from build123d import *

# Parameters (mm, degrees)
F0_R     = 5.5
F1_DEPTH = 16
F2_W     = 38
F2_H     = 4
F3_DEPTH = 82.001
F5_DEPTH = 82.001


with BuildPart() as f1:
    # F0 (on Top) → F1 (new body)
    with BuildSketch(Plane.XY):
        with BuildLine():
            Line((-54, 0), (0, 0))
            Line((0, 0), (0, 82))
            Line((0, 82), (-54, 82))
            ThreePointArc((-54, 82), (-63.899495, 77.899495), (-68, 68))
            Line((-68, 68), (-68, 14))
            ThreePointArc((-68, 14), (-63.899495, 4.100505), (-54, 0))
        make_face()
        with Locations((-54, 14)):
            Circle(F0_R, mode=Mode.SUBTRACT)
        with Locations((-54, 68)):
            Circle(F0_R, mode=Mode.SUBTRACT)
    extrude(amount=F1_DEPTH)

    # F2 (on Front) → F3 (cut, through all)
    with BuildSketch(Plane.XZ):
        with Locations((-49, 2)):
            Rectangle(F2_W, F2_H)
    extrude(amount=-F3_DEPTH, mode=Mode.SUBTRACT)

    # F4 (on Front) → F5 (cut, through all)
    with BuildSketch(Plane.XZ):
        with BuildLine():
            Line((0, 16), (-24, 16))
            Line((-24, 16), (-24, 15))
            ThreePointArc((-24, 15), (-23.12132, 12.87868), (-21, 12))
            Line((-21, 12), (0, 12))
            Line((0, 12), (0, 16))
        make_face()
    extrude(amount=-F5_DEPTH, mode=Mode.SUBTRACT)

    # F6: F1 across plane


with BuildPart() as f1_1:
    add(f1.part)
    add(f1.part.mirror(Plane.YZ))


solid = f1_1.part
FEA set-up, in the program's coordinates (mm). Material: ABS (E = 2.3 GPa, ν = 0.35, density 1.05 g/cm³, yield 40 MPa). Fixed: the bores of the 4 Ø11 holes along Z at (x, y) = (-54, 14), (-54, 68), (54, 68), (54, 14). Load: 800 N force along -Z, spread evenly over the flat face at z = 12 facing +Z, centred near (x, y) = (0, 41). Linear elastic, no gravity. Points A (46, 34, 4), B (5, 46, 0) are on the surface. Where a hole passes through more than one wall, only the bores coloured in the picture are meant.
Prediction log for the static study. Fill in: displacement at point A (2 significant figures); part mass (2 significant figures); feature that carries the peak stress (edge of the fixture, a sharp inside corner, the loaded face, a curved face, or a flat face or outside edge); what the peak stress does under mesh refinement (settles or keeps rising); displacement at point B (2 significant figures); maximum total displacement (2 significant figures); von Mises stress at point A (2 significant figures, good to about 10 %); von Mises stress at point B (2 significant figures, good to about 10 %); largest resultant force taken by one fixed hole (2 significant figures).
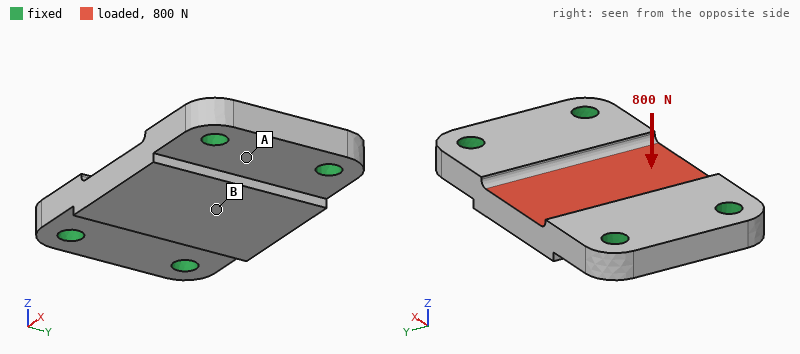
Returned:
0.024 mm
140 g
edge of the fixture
keeps rising
0.15 mm
0.16 mm
1.2 MPa
3.0 MPa
340 N
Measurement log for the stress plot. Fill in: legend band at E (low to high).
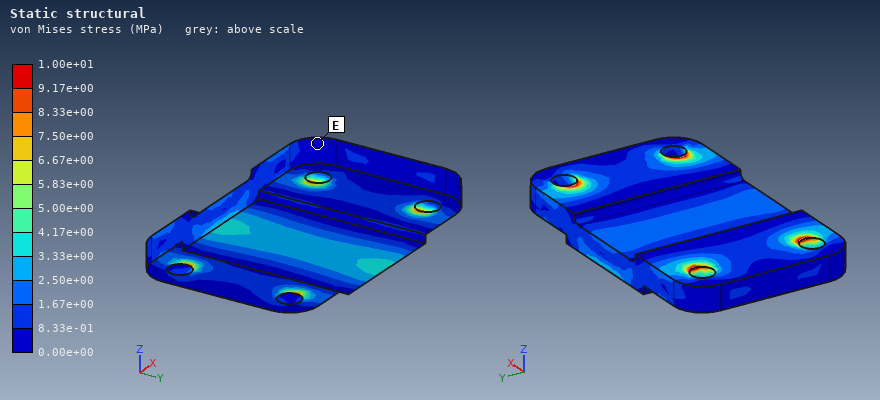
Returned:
0.00e+00 to 8.33e-01 MPa
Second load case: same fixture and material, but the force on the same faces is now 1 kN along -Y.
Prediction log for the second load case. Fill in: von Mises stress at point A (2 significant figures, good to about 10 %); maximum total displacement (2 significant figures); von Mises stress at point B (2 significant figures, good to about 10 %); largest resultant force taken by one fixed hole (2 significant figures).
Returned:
0.80 MPa
53 µm
0.22 MPa
300 N
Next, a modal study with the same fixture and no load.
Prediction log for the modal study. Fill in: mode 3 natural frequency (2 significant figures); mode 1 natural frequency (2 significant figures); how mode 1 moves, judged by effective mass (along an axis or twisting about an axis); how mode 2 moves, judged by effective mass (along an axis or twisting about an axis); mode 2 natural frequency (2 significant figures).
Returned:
3600 Hz
1600 Hz
along Z
twisting about X
2100 Hz
